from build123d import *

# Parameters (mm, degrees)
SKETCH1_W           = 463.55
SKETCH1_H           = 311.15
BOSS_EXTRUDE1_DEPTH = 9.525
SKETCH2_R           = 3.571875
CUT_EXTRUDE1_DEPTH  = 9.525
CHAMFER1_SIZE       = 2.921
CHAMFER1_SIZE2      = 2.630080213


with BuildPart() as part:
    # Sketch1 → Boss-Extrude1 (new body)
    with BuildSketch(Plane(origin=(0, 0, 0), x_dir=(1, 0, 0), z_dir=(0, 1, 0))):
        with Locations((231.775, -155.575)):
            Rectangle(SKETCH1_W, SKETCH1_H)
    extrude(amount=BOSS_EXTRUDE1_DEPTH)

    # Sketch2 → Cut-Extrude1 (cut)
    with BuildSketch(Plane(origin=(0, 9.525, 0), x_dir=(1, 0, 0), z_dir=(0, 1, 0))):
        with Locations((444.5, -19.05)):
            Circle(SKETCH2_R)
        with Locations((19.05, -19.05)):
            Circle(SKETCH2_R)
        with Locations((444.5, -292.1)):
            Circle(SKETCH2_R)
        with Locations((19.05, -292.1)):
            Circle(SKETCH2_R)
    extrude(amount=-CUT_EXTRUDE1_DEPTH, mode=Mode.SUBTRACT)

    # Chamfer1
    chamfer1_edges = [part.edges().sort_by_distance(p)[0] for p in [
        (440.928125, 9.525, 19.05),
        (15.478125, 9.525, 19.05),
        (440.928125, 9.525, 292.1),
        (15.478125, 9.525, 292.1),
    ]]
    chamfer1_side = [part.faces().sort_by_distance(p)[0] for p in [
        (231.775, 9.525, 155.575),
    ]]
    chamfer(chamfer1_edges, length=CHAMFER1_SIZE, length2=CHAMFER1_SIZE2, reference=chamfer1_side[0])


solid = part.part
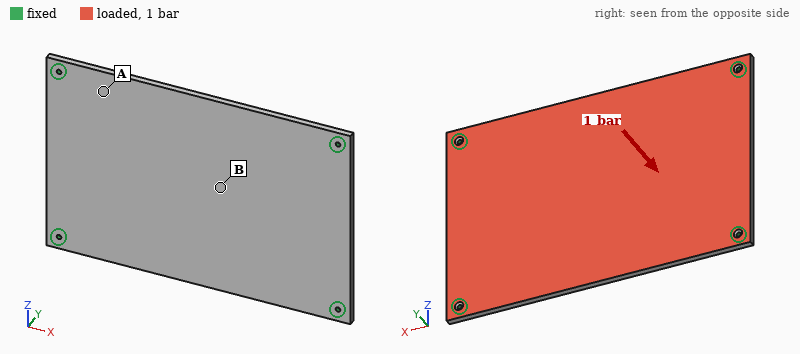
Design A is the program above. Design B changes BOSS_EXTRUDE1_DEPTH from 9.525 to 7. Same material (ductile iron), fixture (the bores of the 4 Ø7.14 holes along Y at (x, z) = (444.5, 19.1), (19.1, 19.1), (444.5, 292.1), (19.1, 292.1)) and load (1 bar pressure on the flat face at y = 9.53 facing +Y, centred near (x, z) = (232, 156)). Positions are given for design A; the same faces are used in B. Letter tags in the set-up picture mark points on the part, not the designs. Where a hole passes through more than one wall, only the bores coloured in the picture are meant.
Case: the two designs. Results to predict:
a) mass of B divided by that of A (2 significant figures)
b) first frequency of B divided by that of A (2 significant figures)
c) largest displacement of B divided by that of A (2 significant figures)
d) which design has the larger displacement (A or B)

0.73
0.74
2.5
B
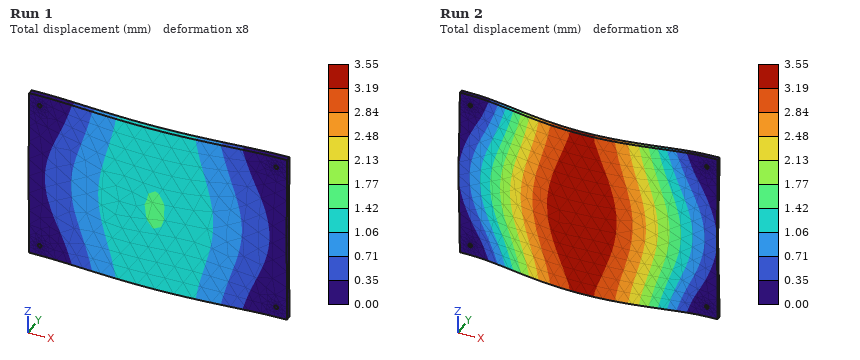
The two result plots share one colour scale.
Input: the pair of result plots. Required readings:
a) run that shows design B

Run 2
